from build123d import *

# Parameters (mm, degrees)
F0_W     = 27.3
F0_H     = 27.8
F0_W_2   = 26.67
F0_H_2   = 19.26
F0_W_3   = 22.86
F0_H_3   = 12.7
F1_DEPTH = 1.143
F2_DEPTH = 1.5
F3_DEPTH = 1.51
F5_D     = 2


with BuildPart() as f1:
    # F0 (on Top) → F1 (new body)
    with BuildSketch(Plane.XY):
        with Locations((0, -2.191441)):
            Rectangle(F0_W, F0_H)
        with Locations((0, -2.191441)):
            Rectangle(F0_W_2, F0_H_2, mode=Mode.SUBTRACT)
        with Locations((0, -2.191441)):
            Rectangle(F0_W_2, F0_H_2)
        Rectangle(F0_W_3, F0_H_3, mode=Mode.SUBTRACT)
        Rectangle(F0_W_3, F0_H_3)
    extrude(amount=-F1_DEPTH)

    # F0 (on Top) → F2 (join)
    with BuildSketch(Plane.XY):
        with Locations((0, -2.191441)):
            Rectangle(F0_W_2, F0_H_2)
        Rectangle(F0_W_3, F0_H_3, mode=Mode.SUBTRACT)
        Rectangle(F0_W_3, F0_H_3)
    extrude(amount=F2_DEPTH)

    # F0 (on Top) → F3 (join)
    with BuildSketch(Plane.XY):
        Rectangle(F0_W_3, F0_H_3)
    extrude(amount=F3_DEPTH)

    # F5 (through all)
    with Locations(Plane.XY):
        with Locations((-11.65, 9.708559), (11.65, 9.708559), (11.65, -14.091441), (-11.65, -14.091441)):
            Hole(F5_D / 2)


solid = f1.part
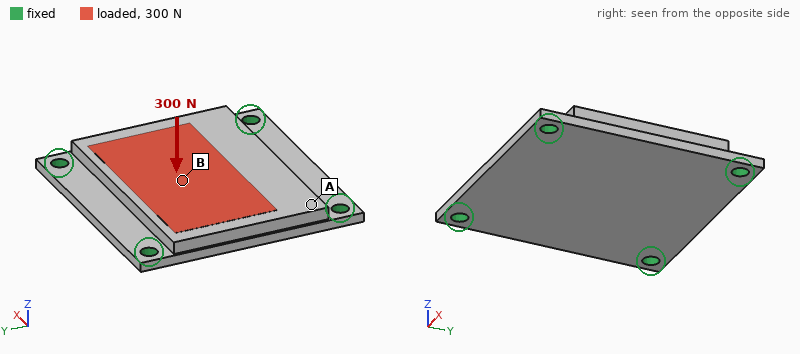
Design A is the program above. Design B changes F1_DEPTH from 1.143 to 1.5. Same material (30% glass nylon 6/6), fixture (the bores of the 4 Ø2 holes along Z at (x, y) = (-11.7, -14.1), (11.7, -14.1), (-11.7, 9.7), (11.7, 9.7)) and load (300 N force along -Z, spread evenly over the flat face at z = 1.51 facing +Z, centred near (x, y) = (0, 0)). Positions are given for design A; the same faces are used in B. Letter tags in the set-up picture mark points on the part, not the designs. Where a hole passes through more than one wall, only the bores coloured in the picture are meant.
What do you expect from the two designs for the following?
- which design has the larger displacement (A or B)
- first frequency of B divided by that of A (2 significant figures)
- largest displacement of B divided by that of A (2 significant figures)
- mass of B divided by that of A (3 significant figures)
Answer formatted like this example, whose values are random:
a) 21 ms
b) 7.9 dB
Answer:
a) A
b) 1.2
c) 0.66
d) 1.16
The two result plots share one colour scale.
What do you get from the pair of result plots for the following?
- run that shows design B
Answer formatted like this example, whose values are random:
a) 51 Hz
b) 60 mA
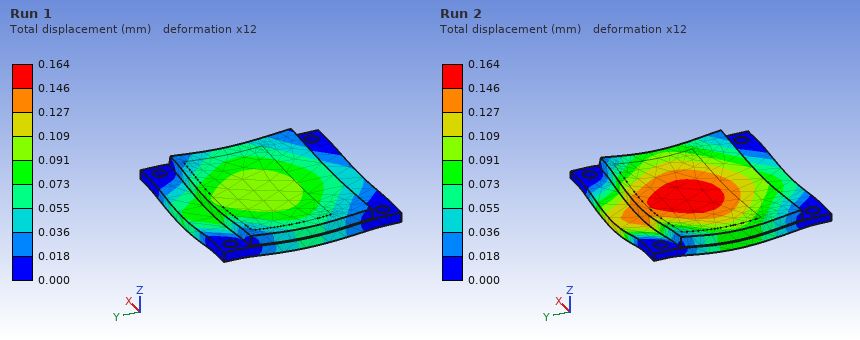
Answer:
a) Run 1
